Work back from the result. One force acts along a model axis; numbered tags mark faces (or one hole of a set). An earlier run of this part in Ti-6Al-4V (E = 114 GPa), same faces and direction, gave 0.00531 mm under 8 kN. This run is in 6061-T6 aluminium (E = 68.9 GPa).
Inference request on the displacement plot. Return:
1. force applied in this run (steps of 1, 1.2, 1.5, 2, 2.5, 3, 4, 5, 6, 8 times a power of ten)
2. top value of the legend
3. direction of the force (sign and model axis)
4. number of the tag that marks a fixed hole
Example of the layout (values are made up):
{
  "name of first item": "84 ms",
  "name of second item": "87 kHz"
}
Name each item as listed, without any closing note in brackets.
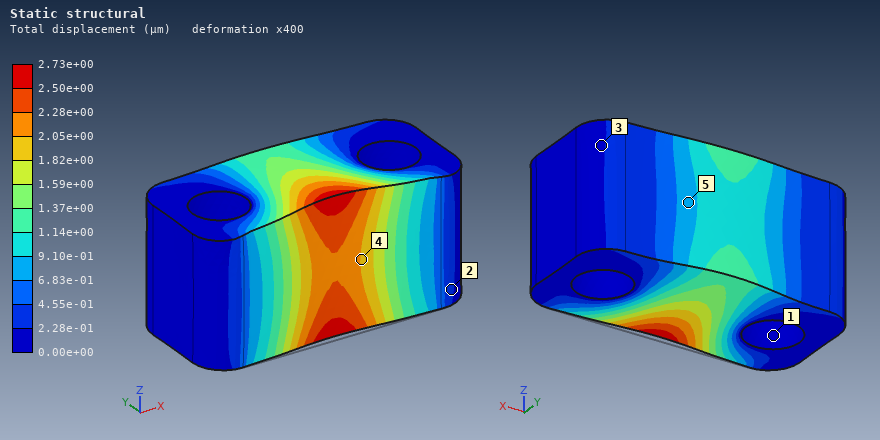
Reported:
{
  "force applied in this run": "2.5 kN",
  "top value of the legend": "2.73e+00 µm",
  "direction of the force": "+Y",
  "number of the tag that marks a fixed hole": "1"
}
